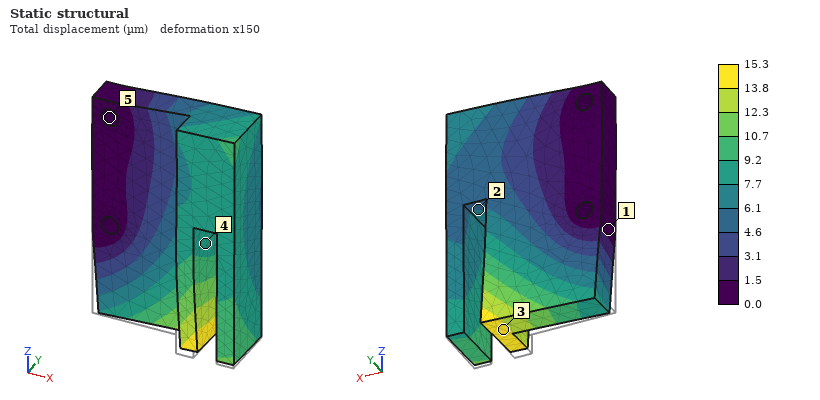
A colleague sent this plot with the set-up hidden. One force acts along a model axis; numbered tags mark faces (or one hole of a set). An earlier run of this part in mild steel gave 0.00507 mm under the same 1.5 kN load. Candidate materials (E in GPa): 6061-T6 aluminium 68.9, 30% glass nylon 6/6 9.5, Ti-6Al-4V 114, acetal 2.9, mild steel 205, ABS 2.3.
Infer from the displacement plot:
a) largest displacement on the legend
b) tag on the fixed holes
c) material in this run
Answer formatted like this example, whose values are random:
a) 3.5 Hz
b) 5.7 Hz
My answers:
a) 15.3 µm
b) 5
c) 6061-T6 aluminium
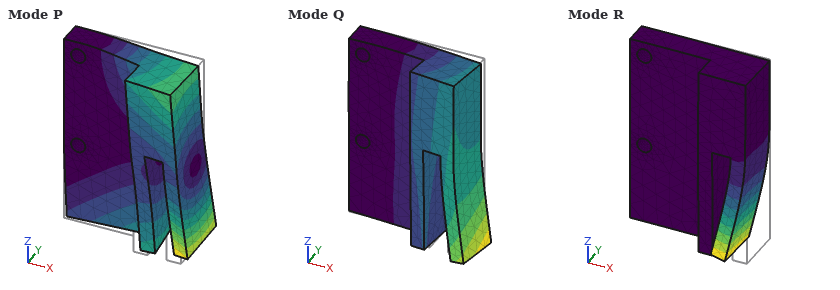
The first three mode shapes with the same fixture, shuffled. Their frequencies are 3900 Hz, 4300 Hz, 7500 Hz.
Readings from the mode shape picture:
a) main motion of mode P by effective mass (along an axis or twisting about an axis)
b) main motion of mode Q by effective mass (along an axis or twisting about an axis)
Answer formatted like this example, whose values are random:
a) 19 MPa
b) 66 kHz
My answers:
a) twisting about X
b) along Y
